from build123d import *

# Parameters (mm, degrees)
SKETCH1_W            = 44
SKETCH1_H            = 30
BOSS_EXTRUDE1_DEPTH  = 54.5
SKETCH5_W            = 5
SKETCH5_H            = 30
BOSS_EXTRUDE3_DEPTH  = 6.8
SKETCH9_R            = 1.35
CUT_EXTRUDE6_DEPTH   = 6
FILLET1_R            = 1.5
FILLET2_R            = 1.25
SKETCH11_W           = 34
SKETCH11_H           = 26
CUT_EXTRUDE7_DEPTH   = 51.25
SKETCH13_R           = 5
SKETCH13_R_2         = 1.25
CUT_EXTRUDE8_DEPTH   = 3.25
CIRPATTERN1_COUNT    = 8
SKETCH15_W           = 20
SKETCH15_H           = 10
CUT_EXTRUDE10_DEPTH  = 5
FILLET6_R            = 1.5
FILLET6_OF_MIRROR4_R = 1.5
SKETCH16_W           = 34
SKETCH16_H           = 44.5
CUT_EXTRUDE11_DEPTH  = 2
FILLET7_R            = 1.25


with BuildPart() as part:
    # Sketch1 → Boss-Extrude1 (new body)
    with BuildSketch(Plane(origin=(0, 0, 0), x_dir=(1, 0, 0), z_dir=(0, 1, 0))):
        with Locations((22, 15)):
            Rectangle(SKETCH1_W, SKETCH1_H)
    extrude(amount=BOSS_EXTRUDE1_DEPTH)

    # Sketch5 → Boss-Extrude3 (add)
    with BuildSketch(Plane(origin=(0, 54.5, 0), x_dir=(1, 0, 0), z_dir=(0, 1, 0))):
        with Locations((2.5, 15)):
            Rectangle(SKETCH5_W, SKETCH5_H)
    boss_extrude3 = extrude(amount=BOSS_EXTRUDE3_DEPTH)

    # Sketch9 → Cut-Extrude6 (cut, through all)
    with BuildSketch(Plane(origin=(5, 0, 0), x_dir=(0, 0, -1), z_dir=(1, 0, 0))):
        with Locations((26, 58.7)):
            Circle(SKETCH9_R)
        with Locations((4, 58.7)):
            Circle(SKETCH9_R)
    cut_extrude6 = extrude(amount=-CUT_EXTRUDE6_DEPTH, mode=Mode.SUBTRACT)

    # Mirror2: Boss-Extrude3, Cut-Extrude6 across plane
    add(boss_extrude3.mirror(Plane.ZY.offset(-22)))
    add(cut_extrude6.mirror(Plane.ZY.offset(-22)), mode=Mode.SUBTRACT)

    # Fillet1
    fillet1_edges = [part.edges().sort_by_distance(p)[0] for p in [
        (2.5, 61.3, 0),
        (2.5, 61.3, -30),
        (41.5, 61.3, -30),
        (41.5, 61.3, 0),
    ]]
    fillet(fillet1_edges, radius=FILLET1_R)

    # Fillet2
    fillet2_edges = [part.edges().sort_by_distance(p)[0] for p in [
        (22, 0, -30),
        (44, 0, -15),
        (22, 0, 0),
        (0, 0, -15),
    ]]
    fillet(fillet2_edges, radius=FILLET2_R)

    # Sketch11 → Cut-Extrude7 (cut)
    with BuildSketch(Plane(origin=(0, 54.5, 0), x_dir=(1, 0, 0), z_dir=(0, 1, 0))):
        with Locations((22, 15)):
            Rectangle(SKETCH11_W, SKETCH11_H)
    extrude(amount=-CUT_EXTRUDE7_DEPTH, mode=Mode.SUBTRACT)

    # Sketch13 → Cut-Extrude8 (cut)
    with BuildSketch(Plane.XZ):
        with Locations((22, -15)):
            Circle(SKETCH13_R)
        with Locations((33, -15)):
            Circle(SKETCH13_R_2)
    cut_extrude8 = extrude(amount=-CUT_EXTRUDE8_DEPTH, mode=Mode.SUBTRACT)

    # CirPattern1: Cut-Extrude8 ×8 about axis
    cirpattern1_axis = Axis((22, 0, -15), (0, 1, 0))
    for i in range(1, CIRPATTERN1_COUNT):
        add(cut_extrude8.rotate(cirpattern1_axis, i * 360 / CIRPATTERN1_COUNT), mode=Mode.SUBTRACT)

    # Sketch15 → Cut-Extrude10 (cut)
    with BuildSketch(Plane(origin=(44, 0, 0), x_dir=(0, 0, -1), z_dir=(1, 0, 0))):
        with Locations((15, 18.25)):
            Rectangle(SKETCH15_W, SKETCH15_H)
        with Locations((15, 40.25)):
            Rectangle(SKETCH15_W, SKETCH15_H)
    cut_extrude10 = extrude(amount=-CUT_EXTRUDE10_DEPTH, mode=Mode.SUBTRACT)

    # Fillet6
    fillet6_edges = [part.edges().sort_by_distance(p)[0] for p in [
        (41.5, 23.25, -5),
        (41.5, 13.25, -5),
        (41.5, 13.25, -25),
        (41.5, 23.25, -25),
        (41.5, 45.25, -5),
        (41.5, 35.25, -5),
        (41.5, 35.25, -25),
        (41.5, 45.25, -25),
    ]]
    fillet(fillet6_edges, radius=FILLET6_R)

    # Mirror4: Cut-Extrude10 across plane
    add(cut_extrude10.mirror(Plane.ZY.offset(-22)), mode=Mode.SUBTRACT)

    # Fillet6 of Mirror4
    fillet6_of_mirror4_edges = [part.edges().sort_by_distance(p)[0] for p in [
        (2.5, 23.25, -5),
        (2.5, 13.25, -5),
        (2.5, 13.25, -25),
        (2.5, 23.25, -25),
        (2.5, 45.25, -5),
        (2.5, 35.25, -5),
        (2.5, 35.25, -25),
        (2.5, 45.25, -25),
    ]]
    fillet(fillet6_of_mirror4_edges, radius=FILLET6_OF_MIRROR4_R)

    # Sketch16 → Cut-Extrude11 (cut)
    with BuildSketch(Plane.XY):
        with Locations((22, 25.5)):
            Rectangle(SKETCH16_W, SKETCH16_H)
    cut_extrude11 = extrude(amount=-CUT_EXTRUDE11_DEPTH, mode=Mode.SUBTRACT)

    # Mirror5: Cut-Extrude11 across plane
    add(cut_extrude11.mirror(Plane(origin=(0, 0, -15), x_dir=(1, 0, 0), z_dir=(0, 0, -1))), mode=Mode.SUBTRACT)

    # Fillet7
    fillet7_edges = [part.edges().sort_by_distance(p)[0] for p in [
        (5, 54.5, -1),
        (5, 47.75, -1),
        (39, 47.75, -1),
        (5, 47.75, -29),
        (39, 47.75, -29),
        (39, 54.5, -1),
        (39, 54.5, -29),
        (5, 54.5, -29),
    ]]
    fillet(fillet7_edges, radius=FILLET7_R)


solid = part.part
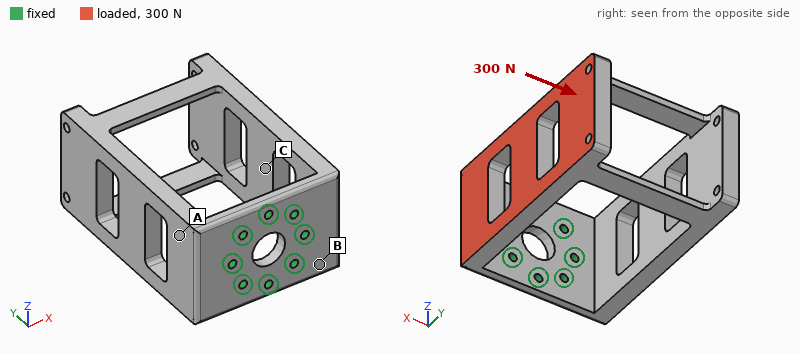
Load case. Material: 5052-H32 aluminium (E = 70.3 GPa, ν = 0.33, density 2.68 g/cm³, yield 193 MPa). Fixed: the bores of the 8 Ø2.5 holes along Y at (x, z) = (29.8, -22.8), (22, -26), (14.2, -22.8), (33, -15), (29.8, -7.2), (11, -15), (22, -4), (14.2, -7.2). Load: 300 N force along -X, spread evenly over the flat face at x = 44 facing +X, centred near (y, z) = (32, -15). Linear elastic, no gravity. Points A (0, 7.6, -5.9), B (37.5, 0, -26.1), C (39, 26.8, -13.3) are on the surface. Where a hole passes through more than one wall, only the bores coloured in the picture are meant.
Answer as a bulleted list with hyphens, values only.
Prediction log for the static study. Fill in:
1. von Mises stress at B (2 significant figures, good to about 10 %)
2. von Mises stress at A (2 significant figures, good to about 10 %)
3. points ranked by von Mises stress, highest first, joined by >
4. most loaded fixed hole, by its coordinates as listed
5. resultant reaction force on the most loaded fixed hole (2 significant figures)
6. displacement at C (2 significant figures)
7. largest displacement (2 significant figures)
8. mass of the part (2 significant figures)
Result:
- 49 MPa
- 17 MPa
- B > A > C
- (33, -15)
- 270 N
- 0.15 mm
- 0.28 mm
- 49 g
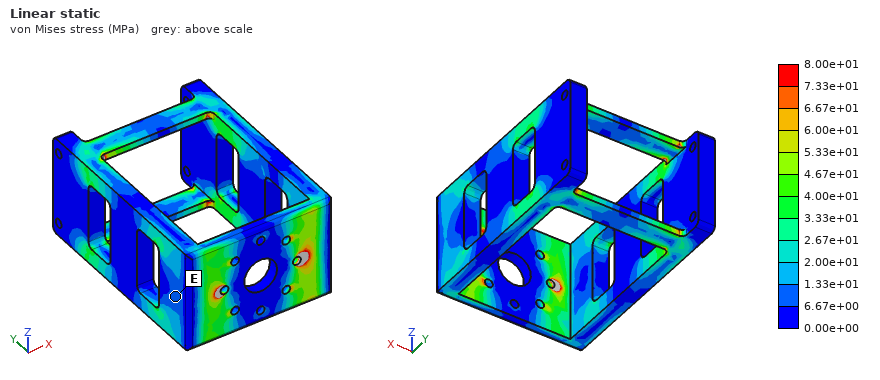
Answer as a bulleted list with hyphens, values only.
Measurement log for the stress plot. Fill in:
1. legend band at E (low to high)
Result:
- 6.67e+00 to 1.33e+01 MPa
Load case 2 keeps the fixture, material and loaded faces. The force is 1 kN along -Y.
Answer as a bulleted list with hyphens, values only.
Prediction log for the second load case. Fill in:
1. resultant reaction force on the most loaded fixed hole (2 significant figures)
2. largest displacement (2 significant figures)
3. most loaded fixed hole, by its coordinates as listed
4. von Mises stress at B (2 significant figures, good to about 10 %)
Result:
- 880 N
- 0.23 mm
- (33, -15)
- 40 MPa
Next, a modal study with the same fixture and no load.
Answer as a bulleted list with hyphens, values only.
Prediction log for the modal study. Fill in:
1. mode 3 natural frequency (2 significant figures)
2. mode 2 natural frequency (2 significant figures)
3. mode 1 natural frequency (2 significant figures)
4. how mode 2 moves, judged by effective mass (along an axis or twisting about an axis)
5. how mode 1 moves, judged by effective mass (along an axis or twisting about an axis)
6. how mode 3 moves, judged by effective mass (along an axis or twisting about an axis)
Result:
- 1900 Hz
- 1500 Hz
- 920 Hz
- along Z
- along X
- twisting about Y
